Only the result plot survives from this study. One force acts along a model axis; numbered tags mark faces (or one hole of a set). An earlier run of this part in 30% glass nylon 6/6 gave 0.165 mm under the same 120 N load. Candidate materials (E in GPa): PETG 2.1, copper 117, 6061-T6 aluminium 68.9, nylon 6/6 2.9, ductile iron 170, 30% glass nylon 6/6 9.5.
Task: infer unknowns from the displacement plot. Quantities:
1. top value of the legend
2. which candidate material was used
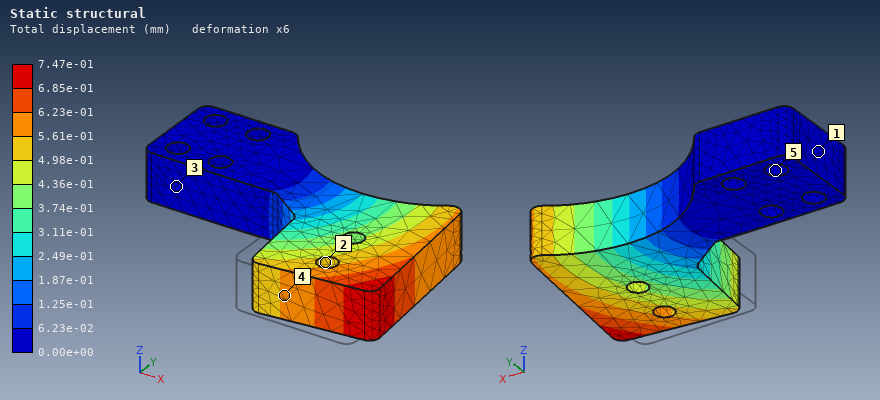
7.47e-01 mm
PETG
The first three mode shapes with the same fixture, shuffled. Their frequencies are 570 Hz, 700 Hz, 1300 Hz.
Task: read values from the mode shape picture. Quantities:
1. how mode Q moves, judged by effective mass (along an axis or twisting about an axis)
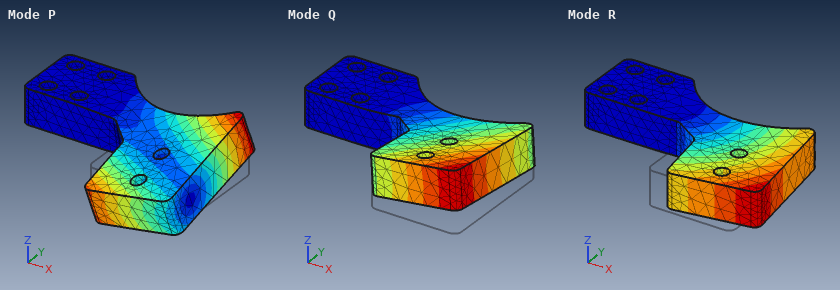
along Z
